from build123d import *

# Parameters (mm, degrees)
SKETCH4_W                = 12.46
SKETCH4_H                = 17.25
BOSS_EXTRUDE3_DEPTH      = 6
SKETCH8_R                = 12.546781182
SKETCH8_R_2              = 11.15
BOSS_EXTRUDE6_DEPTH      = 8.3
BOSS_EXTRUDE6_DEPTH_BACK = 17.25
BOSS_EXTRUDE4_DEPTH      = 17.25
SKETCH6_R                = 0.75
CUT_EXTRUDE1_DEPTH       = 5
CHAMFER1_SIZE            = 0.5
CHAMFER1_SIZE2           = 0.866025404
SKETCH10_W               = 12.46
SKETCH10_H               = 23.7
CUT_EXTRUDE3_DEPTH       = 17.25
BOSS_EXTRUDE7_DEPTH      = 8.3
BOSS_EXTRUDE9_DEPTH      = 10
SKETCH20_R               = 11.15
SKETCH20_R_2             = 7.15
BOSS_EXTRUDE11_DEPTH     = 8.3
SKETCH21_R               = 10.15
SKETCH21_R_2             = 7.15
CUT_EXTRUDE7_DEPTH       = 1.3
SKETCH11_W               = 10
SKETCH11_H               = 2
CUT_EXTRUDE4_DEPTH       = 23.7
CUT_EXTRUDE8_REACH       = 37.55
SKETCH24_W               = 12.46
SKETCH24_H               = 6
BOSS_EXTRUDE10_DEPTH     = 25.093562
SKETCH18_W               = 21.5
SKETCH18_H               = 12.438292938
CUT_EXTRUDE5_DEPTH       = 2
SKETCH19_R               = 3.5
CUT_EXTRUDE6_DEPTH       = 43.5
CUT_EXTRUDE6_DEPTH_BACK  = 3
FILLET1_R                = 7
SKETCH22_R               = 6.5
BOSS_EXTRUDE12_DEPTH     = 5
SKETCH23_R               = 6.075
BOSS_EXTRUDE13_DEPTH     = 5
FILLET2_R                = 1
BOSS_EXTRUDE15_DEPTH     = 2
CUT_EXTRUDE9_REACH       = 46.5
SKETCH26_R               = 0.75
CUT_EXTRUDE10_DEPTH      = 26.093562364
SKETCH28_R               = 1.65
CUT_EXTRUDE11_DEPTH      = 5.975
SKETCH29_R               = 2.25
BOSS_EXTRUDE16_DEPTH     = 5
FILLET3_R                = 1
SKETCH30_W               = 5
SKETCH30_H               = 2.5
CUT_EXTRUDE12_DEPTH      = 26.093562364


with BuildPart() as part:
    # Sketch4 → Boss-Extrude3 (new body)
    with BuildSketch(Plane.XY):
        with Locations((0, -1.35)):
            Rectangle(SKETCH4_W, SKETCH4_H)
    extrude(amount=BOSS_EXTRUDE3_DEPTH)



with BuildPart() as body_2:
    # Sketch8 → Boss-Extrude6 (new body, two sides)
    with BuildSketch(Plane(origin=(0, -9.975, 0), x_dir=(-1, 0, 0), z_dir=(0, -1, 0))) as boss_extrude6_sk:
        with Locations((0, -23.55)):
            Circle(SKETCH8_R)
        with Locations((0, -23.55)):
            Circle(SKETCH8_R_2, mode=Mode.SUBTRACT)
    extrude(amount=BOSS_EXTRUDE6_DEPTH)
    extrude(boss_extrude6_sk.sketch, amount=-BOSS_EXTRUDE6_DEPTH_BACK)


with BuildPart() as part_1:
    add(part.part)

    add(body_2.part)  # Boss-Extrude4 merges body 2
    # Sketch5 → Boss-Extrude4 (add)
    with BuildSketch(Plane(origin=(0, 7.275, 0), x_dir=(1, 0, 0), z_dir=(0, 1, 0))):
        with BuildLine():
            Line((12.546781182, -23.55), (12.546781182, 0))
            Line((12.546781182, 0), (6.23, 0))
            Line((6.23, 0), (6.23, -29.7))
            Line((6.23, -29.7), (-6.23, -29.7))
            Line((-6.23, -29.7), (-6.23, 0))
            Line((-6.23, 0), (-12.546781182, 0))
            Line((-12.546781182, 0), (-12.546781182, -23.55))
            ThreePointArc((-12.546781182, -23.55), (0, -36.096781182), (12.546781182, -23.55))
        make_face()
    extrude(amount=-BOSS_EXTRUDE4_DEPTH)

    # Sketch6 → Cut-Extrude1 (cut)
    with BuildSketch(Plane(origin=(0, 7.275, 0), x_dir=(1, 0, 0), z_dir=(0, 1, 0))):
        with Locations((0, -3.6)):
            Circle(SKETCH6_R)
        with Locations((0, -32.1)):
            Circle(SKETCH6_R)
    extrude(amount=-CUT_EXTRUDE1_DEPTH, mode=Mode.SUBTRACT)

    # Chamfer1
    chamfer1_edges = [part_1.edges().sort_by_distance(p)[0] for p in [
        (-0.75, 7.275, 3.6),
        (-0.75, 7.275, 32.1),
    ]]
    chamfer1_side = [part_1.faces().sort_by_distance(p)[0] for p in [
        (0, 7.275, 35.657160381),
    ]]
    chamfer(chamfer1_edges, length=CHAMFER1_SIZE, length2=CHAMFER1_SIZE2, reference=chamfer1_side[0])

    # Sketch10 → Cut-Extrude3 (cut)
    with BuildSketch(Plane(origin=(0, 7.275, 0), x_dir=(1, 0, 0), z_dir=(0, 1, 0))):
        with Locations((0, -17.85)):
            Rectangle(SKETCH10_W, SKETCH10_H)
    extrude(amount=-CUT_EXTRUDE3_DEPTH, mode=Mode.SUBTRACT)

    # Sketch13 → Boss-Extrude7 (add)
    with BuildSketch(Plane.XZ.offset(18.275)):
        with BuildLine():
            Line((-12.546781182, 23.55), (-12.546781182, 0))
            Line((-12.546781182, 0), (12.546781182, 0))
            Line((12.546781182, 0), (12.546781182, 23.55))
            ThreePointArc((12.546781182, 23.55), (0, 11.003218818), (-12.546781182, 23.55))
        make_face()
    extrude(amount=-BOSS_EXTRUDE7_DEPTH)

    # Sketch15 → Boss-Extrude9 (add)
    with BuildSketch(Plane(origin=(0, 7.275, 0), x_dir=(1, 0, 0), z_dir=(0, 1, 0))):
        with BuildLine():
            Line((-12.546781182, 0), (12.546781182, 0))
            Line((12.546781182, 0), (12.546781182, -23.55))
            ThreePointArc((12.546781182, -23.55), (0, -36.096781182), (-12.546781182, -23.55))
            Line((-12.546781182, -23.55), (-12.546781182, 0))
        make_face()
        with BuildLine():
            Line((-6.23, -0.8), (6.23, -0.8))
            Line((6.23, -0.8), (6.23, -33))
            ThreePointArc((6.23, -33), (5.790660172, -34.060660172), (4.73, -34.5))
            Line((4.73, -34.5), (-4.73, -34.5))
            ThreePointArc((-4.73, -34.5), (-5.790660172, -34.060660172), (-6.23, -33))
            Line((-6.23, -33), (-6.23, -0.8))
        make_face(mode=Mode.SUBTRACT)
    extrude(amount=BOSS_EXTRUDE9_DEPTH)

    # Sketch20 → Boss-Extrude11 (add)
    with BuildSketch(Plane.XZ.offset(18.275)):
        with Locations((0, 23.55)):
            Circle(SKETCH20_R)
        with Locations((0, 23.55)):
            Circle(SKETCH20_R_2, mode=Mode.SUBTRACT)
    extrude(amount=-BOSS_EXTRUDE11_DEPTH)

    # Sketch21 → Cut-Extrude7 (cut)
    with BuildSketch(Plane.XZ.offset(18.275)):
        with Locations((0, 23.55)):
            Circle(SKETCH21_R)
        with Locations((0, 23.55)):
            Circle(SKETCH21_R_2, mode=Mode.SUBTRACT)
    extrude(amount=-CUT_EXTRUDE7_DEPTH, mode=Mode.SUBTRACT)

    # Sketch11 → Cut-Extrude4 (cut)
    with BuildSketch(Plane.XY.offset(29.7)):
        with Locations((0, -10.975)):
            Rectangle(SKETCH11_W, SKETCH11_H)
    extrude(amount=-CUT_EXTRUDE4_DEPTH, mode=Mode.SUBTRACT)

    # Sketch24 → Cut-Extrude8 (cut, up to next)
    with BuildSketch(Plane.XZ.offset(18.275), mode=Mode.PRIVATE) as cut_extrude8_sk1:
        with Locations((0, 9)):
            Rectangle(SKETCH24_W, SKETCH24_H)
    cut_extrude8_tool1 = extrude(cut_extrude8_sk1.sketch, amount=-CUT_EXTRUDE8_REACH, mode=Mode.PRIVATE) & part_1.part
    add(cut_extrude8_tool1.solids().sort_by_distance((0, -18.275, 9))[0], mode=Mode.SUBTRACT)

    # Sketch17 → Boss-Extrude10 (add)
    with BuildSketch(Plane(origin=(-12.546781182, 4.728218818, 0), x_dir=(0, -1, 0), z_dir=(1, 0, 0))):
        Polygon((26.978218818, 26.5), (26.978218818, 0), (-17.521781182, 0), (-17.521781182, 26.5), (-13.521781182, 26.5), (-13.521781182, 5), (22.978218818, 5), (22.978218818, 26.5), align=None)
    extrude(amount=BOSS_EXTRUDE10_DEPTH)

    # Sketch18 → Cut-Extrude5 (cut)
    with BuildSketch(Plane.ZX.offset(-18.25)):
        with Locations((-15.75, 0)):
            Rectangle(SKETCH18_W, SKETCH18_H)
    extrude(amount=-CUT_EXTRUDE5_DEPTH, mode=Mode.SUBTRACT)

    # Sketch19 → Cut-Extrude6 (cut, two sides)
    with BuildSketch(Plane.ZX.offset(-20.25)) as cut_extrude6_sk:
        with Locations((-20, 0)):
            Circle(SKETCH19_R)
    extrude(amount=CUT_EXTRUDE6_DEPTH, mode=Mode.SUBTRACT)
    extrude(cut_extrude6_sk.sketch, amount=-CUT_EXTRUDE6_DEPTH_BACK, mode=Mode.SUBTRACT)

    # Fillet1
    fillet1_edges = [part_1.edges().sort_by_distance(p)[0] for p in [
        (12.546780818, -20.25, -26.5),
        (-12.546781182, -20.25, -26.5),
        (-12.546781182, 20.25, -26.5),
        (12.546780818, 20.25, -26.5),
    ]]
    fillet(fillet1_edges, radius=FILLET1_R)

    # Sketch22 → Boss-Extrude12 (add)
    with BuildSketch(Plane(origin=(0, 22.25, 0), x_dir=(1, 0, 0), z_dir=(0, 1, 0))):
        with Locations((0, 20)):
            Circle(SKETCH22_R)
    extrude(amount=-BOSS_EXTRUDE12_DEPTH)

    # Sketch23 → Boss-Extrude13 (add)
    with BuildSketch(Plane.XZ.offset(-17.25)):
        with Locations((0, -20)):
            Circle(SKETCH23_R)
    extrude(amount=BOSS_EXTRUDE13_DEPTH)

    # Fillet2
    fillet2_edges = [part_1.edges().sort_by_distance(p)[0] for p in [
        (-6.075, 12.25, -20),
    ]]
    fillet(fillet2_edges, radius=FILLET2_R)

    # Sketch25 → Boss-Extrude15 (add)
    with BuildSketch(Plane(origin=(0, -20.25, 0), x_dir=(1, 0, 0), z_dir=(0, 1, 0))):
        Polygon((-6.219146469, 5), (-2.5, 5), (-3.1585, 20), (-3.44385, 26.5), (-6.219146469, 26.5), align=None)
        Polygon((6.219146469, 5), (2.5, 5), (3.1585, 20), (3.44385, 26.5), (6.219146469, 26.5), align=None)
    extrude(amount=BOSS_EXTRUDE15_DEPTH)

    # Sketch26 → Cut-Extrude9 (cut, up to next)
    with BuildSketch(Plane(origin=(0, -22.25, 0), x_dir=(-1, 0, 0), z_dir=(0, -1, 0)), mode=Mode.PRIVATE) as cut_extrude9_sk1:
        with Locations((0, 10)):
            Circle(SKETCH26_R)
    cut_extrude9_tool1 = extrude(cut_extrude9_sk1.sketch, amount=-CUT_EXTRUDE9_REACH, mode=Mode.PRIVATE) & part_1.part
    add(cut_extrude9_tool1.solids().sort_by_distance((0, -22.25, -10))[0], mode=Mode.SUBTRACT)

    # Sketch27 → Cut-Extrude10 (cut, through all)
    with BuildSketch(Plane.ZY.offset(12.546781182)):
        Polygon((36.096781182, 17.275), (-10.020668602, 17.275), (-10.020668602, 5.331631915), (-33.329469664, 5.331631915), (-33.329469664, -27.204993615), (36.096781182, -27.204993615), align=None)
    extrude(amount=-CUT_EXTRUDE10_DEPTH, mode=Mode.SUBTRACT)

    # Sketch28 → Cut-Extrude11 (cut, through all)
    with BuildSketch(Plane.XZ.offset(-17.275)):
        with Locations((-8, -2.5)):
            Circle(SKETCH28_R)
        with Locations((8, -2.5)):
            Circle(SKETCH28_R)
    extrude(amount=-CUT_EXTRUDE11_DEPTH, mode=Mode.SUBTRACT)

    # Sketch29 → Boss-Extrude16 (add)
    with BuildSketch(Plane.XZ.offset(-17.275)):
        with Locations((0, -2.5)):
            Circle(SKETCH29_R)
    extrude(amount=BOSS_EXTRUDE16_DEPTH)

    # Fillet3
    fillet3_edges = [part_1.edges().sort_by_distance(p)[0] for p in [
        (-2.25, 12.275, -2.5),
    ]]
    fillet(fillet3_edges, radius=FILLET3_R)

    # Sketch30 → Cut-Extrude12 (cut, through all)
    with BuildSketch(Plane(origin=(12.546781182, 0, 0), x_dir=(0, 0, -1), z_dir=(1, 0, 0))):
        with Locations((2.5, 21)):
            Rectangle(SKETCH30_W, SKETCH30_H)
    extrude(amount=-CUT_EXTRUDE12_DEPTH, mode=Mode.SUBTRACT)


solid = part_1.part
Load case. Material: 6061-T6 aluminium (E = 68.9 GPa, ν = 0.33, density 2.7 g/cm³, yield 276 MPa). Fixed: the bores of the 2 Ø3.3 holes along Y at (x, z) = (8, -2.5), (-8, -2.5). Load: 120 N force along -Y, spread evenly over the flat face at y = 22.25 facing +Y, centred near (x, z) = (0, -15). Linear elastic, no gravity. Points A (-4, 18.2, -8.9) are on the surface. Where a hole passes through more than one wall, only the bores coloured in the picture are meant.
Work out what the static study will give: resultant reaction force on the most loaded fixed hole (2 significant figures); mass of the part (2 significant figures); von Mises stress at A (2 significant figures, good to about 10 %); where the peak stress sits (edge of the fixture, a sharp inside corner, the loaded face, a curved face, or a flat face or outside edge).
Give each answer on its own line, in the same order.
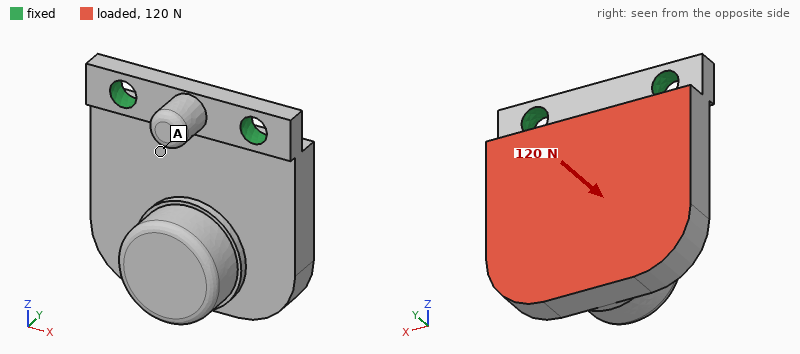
63 N
8.4 g
13 MPa
a flat face or outside edge
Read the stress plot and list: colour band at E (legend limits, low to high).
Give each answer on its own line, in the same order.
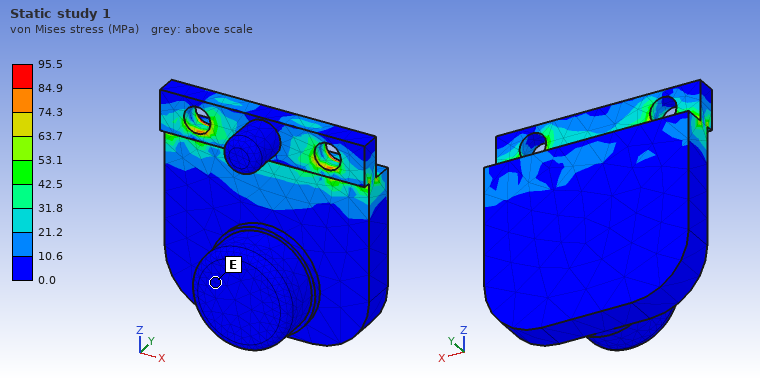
0.0 to 10.6 MPa
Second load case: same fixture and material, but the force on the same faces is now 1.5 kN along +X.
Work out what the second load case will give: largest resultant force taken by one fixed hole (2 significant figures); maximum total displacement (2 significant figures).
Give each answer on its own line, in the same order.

1.3 kN
30 µm
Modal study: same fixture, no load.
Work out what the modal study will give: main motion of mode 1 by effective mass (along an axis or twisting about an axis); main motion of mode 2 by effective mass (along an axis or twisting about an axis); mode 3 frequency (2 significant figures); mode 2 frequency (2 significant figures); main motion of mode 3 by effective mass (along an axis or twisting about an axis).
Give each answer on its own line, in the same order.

along Y
along X
17 kHz
9700 Hz
along X
